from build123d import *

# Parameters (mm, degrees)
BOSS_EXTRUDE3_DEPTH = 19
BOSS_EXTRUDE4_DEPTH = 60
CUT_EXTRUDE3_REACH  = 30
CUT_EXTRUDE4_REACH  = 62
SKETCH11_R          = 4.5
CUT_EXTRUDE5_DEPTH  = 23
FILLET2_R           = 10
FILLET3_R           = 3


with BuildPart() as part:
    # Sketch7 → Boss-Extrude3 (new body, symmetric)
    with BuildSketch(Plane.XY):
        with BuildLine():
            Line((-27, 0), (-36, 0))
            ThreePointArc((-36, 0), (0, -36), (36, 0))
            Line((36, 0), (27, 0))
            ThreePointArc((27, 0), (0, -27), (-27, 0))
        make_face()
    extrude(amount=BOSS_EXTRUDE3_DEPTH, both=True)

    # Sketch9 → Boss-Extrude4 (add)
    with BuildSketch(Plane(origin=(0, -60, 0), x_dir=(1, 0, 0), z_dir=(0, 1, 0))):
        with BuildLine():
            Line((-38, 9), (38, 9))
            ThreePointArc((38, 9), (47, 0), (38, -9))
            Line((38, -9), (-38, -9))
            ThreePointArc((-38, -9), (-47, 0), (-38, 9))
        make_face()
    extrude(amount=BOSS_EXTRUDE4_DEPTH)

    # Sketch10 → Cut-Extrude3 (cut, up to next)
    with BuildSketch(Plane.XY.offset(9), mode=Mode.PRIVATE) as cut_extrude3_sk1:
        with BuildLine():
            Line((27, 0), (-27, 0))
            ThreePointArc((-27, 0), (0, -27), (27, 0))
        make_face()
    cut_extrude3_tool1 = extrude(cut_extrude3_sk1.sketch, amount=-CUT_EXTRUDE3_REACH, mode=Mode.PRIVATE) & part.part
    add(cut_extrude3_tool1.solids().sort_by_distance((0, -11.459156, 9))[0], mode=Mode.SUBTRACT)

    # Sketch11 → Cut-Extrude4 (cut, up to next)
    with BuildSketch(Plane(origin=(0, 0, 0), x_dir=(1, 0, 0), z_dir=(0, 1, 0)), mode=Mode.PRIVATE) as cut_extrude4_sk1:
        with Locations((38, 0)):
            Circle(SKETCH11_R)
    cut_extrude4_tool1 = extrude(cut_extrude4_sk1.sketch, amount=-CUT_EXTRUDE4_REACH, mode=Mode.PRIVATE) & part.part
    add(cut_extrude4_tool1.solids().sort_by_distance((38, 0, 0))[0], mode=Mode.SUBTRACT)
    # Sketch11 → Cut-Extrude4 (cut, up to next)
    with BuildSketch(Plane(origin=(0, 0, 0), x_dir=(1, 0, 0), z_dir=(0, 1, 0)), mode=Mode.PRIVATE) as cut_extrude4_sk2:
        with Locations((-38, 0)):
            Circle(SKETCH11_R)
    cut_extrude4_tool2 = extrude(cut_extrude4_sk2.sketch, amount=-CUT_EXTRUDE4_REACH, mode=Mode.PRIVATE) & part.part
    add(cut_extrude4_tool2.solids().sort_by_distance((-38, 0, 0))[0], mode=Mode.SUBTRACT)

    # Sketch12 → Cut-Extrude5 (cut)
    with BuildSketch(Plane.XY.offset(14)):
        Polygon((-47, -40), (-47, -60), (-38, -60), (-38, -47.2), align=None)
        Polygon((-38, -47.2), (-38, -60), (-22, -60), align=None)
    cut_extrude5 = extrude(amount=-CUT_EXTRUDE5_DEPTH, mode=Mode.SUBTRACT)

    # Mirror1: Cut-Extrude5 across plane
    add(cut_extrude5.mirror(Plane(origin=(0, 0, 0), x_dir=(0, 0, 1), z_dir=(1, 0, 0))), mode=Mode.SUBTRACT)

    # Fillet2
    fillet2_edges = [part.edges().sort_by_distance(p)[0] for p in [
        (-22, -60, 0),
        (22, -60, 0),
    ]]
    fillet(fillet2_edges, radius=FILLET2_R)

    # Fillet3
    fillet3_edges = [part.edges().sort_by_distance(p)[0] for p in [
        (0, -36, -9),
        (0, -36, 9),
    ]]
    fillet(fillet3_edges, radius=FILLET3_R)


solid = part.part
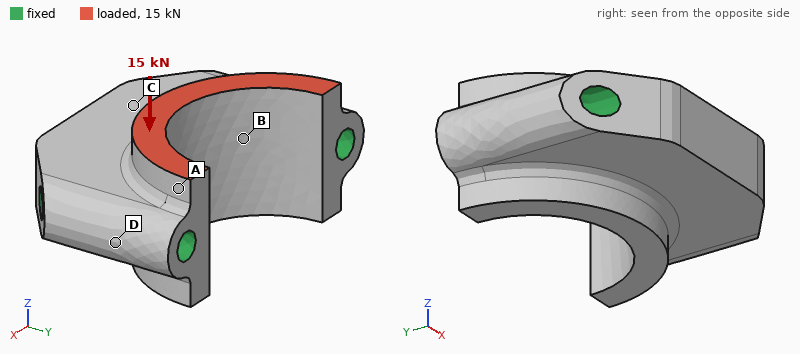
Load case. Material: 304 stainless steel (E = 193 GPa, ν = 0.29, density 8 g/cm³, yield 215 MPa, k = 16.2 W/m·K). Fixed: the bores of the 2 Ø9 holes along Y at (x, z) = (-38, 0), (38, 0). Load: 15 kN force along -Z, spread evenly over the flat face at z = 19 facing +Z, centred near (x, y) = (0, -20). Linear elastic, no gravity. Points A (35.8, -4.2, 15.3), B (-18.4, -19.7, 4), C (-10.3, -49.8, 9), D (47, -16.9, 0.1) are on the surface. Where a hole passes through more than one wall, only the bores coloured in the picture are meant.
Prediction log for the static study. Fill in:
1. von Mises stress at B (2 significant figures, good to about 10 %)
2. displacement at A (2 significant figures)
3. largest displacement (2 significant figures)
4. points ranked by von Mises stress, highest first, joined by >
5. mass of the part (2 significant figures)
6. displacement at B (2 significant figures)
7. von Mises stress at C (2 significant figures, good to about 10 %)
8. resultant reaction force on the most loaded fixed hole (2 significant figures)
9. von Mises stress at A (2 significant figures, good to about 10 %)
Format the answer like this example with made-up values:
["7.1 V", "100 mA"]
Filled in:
["13 MPa", "2.2 µm", "5.5 µm", "A > B > C > D", "650 g", "3.3 µm", "8.9 MPa", "7.5 kN", "17 MPa"]
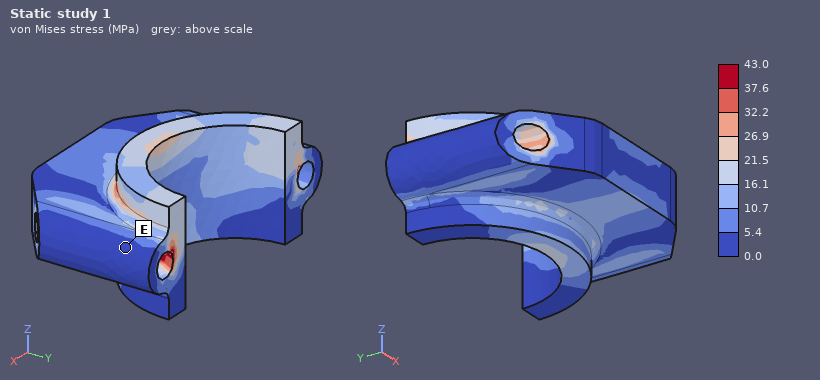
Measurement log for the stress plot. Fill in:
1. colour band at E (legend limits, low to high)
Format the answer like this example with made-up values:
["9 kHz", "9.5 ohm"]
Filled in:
["0.0 to 5.4 MPa"]
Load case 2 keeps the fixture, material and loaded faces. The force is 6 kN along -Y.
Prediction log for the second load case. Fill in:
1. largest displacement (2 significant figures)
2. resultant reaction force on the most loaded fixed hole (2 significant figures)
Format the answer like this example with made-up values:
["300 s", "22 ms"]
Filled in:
["5.9 µm", "3.1 kN"]
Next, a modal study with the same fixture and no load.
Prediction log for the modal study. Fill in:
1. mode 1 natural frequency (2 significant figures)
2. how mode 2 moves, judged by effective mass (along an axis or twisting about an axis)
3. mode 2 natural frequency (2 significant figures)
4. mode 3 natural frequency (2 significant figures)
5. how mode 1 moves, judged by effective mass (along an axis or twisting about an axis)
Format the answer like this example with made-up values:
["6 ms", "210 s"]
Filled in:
["11 kHz", "along Y", "18 kHz", "19 kHz", "along Z"]
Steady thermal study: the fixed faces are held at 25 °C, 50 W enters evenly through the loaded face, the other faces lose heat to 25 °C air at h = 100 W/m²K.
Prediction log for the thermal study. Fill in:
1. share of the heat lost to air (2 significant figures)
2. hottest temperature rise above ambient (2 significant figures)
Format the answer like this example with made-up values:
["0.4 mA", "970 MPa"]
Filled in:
["32 %", "60 K"]
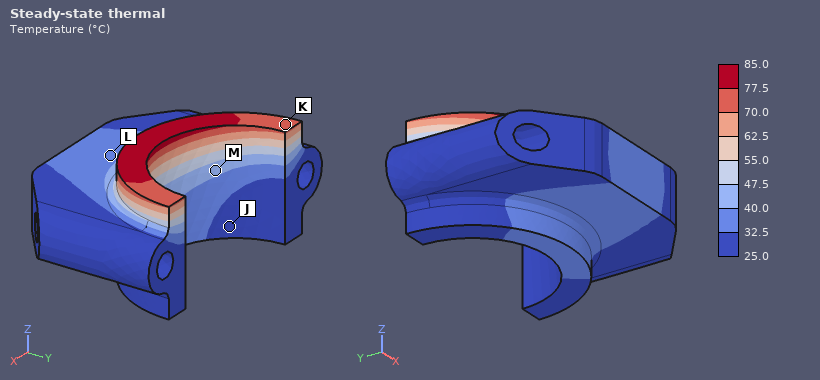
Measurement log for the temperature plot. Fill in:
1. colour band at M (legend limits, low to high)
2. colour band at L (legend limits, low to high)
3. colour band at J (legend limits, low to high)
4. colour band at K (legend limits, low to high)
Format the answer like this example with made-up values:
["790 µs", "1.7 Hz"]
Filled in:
["40.0 to 47.5 °C", "32.5 to 40.0 °C", "25.0 to 32.5 °C", "70.0 to 77.5 °C"]
